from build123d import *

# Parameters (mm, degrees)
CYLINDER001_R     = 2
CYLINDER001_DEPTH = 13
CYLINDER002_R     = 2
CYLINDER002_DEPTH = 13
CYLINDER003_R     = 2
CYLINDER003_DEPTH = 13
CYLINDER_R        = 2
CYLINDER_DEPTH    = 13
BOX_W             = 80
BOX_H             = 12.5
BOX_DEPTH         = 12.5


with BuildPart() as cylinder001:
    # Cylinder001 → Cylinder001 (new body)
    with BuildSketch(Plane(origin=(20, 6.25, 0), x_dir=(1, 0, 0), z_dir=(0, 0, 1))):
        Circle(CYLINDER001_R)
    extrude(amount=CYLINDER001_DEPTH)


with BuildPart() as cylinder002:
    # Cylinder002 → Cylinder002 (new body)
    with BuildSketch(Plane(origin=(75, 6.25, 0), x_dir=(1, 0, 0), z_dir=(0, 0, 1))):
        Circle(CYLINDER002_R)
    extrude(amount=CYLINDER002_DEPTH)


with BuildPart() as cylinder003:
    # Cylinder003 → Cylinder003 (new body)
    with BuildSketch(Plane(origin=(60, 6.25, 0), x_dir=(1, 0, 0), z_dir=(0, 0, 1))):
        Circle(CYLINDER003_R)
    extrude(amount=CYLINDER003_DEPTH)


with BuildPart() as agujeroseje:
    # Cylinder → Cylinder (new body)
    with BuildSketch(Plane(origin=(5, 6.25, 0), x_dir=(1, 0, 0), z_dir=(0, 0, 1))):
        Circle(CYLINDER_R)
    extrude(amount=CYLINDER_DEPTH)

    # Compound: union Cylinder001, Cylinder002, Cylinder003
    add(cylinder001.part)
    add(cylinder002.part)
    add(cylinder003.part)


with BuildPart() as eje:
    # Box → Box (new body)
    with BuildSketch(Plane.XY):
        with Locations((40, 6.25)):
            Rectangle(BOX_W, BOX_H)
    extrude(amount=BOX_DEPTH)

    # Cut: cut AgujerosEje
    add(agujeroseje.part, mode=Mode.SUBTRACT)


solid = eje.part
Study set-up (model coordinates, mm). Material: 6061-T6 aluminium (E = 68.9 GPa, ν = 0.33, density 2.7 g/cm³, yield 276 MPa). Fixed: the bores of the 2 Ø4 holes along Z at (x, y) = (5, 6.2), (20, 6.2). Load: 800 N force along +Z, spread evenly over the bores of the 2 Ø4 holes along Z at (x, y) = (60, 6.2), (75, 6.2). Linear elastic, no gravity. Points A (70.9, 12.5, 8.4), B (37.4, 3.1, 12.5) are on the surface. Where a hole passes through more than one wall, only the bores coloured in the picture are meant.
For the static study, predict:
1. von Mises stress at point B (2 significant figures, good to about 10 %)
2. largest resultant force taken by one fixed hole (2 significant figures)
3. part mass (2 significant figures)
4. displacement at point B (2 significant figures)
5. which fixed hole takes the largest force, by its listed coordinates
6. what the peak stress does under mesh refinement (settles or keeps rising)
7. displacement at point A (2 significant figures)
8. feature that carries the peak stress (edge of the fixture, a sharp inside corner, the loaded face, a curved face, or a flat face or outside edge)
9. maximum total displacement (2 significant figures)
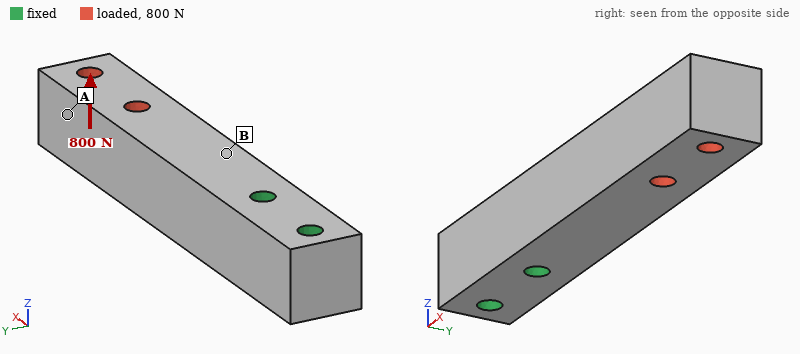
74 MPa
1.1 kN
32 g
0.047 mm
(20, 6.2)
keeps rising
0.24 mm
edge of the fixture
0.30 mm
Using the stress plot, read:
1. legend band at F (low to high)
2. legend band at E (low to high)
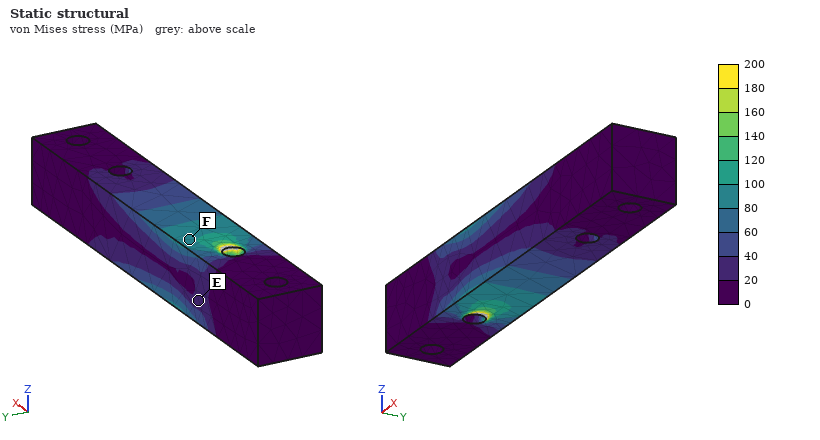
80 to 100 MPa
20 to 40 MPa
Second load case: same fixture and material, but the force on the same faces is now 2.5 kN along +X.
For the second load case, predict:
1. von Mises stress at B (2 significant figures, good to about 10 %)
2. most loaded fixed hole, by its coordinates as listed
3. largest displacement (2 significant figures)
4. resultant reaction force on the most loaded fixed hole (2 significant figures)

16 MPa
(20, 6.2)
13 µm
2.3 kN
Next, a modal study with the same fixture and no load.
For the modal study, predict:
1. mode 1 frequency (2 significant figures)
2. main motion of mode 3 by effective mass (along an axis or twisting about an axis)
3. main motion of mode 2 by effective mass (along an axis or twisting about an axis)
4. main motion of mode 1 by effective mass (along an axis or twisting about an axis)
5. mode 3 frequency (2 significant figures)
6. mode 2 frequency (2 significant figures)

2600 Hz
twisting about X
along Z
along Y
12 kHz
2800 Hz
